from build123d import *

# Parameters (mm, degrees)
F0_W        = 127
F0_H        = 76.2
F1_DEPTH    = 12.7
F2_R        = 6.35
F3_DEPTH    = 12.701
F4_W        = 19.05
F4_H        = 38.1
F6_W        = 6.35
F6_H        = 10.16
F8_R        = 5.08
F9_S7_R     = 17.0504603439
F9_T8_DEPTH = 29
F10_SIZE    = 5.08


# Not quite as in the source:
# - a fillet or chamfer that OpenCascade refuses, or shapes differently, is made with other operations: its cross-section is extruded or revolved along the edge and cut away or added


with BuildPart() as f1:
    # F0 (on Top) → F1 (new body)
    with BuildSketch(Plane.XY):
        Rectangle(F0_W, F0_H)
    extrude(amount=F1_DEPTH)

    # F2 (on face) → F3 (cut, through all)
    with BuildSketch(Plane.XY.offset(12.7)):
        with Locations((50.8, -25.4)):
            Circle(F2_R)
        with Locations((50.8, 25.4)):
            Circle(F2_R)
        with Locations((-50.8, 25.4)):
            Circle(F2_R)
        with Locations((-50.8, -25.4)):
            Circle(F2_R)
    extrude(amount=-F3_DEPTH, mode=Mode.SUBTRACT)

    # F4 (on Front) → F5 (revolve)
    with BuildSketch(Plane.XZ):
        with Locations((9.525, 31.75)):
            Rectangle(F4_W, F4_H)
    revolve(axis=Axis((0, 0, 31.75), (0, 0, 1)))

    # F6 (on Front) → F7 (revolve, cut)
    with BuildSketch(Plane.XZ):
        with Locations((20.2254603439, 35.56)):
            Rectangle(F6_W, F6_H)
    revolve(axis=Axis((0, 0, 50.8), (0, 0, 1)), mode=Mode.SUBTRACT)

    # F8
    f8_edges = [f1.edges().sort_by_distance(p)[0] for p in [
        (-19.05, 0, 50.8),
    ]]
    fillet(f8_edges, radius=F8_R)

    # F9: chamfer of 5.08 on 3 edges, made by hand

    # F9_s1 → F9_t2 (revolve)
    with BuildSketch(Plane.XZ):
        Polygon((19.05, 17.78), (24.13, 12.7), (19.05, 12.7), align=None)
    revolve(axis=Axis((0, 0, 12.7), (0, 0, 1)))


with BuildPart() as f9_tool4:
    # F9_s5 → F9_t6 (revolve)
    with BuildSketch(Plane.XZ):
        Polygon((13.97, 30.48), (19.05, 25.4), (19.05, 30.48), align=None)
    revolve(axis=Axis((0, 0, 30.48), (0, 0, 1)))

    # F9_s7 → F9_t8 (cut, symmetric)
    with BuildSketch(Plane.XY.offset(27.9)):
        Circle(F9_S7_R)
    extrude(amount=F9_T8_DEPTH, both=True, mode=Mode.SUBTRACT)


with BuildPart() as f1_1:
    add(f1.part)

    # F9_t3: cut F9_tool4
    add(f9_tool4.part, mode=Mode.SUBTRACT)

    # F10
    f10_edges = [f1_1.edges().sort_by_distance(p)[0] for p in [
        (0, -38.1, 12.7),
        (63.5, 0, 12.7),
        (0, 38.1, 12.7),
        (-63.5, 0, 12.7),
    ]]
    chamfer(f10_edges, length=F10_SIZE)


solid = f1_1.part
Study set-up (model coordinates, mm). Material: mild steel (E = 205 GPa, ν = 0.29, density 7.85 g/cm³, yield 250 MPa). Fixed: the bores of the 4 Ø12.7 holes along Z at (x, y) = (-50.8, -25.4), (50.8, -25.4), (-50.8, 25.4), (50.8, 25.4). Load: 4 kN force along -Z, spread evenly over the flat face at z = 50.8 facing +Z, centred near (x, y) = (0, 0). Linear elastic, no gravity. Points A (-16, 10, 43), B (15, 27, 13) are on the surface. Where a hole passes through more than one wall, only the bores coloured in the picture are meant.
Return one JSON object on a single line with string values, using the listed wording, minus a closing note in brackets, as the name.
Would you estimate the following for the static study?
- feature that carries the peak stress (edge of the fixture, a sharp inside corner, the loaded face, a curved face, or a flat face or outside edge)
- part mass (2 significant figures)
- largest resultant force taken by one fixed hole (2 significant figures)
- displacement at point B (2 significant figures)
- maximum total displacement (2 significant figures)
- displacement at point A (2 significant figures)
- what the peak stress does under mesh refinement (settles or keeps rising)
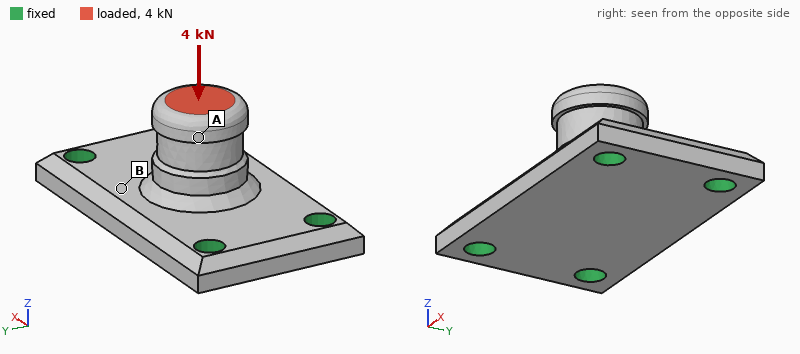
{"feature that carries the peak stress": "edge of the fixture", "part mass": "1.2 kg", "largest resultant force taken by one fixed hole": "1.1 kN", "displacement at point B": "4.2 µm", "maximum total displacement": "5.8 µm", "displacement at point A": "5.5 µm", "what the peak stress does under mesh refinement": "keeps rising"}
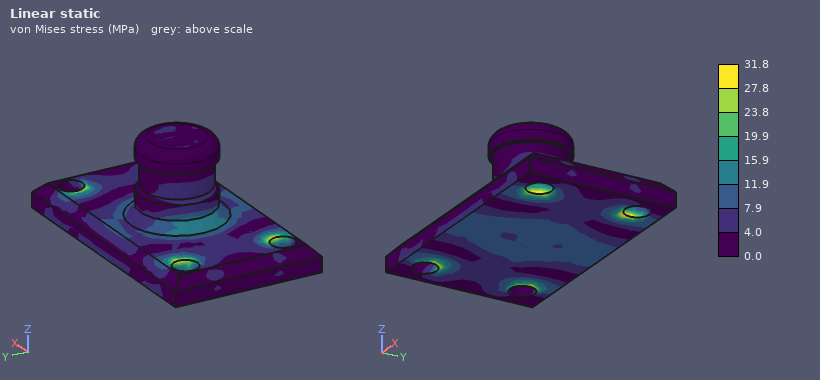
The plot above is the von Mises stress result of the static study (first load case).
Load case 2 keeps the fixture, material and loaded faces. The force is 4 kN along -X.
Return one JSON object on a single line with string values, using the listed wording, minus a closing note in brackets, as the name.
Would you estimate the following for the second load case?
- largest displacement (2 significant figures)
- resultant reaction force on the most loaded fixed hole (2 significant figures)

{"largest displacement": "15 µm", "resultant reaction force on the most loaded fixed hole": "1.6 kN"}
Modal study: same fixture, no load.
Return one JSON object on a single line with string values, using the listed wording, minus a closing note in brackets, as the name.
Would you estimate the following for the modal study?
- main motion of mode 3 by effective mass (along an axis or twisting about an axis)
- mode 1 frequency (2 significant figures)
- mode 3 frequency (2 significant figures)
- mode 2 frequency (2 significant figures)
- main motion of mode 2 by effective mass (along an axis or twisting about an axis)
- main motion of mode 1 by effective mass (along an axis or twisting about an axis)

{"main motion of mode 3 by effective mass": "along X", "mode 1 frequency": "5100 Hz", "mode 3 frequency": "7500 Hz", "mode 2 frequency": "5400 Hz", "main motion of mode 2 by effective mass": "along Z", "main motion of mode 1 by effective mass": "along Y"}
